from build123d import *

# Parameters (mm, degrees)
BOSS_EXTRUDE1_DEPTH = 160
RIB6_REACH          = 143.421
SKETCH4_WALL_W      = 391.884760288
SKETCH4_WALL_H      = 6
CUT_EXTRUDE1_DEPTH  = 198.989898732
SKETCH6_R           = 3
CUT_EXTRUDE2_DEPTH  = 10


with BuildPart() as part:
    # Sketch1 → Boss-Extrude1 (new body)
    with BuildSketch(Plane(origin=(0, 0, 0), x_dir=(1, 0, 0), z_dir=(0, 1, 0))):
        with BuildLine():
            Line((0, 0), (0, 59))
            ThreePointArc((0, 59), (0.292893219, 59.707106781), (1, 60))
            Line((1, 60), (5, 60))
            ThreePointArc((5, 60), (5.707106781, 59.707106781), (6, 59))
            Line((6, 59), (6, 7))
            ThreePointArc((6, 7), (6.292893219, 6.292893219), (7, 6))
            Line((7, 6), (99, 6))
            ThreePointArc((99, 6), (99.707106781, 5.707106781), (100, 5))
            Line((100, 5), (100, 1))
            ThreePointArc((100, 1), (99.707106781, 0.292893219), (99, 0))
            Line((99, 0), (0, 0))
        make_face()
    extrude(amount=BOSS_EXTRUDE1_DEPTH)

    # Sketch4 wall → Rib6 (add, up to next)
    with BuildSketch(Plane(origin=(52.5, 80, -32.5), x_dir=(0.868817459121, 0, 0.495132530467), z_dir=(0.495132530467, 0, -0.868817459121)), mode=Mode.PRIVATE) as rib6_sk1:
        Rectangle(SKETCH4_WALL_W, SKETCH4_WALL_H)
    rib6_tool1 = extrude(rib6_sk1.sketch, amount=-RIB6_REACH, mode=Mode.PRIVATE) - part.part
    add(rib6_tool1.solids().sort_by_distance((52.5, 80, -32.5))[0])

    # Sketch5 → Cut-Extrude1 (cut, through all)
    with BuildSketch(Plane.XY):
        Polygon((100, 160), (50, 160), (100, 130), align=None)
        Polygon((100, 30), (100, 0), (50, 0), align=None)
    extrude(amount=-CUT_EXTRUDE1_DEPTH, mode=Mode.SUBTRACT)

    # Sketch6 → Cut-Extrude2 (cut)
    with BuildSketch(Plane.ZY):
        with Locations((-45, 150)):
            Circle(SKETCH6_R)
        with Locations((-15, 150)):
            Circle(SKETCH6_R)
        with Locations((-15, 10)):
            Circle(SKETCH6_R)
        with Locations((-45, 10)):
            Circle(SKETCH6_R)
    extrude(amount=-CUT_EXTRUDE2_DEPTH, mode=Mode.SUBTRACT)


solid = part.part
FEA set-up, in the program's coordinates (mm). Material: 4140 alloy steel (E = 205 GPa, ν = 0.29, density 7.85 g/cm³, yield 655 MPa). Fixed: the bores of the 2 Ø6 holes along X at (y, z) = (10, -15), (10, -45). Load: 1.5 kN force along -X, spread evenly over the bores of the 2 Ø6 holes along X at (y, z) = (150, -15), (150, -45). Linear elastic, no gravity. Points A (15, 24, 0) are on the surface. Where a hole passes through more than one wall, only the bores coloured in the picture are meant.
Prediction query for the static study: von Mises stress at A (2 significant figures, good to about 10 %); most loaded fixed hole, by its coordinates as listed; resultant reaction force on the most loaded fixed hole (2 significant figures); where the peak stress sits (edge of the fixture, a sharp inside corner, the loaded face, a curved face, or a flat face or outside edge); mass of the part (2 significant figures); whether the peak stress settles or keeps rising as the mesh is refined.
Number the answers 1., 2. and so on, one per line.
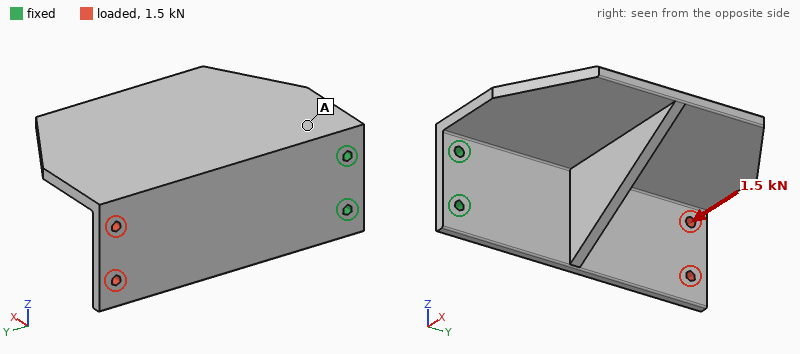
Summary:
1. 66 MPa
2. (10, -15)
3. 1.1 kN
4. edge of the fixture
5. 1.2 kg
6. keeps rising
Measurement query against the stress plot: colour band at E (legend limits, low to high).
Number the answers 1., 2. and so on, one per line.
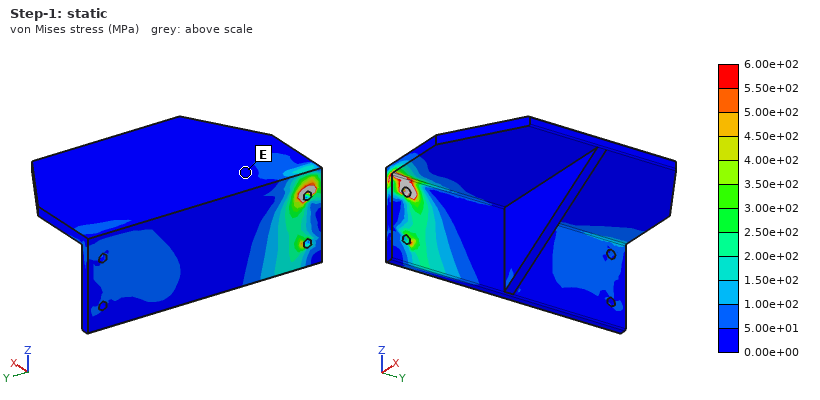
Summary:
1. 0.00e+00 to 5.00e+01 MPa
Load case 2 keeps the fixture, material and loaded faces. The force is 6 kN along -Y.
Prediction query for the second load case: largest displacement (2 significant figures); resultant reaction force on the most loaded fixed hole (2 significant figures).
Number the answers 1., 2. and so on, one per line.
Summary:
1. 18 µm
2. 3.0 kN
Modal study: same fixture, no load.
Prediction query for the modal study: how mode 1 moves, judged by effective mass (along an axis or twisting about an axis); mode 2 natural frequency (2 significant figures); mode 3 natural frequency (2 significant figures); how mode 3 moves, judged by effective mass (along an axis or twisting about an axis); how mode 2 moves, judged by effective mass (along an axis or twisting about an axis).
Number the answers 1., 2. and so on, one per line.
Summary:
1. along X
2. 380 Hz
3. 1100 Hz
4. twisting about X
5. along Z
